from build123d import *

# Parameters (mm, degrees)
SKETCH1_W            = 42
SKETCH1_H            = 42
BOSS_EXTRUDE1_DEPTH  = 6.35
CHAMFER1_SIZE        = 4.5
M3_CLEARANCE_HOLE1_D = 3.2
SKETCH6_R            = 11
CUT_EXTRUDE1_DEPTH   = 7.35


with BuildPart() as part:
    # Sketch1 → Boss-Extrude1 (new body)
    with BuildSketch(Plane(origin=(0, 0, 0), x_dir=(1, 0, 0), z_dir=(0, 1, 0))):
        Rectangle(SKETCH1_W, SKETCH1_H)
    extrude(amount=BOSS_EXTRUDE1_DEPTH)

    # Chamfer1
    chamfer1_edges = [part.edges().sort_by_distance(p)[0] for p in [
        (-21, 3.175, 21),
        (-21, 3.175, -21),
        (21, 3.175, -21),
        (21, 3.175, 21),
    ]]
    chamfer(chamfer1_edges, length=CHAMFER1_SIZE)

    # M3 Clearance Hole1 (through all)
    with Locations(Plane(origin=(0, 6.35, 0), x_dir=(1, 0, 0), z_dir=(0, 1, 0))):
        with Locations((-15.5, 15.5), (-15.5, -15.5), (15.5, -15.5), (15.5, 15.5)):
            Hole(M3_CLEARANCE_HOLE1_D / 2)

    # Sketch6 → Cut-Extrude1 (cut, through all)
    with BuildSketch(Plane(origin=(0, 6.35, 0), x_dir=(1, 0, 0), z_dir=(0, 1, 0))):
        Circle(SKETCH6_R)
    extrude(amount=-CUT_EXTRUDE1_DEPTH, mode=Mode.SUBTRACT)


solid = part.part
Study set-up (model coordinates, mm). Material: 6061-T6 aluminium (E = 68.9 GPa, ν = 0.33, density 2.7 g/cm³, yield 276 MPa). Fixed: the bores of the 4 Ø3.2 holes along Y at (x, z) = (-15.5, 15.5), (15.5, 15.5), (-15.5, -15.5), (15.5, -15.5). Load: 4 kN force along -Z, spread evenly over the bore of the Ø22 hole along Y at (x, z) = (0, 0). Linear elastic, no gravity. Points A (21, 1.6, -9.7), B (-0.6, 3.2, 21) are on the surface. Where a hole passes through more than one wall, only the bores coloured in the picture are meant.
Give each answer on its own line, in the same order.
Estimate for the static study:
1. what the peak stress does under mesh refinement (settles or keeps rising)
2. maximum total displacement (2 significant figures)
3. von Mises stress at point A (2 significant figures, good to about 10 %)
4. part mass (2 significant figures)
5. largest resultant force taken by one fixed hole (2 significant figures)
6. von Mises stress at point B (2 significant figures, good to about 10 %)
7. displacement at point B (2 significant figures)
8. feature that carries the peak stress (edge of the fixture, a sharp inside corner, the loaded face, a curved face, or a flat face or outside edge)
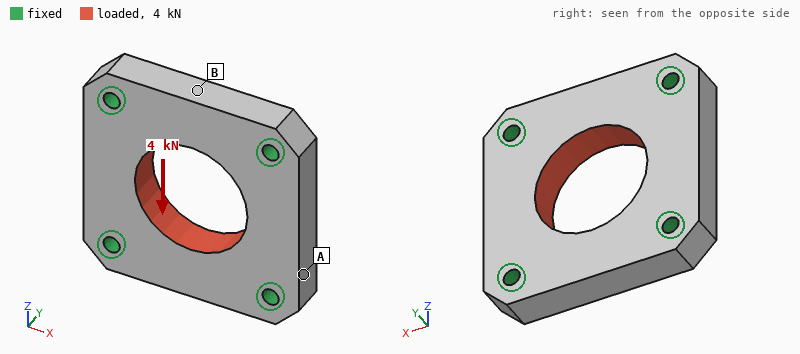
keeps rising
6.0 µm
7.3 MPa
22 g
1.0 kN
18 MPa
5.1 µm
edge of the fixture
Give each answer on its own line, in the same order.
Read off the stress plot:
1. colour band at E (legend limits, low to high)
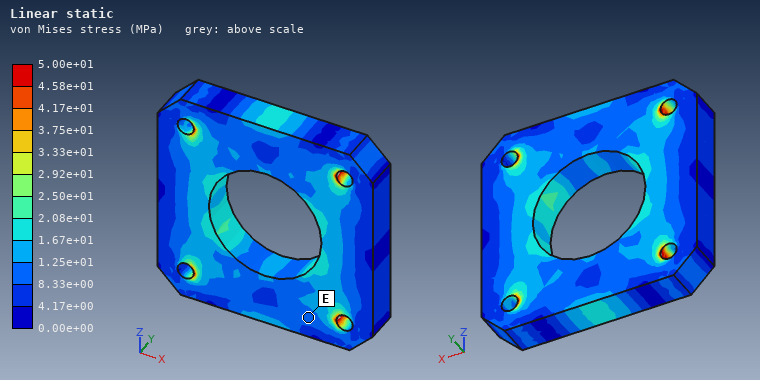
8.33e+00 to 1.25e+01 MPa
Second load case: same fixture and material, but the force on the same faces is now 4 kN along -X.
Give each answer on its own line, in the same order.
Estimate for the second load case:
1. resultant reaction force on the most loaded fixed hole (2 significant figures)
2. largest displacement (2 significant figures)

1.0 kN
6.0 µm
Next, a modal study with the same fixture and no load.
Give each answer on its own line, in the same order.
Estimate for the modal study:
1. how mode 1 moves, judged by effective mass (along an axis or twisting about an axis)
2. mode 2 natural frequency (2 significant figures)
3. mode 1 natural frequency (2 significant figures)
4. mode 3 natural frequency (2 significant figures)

along Y
28 kHz
26 kHz
29 kHz
